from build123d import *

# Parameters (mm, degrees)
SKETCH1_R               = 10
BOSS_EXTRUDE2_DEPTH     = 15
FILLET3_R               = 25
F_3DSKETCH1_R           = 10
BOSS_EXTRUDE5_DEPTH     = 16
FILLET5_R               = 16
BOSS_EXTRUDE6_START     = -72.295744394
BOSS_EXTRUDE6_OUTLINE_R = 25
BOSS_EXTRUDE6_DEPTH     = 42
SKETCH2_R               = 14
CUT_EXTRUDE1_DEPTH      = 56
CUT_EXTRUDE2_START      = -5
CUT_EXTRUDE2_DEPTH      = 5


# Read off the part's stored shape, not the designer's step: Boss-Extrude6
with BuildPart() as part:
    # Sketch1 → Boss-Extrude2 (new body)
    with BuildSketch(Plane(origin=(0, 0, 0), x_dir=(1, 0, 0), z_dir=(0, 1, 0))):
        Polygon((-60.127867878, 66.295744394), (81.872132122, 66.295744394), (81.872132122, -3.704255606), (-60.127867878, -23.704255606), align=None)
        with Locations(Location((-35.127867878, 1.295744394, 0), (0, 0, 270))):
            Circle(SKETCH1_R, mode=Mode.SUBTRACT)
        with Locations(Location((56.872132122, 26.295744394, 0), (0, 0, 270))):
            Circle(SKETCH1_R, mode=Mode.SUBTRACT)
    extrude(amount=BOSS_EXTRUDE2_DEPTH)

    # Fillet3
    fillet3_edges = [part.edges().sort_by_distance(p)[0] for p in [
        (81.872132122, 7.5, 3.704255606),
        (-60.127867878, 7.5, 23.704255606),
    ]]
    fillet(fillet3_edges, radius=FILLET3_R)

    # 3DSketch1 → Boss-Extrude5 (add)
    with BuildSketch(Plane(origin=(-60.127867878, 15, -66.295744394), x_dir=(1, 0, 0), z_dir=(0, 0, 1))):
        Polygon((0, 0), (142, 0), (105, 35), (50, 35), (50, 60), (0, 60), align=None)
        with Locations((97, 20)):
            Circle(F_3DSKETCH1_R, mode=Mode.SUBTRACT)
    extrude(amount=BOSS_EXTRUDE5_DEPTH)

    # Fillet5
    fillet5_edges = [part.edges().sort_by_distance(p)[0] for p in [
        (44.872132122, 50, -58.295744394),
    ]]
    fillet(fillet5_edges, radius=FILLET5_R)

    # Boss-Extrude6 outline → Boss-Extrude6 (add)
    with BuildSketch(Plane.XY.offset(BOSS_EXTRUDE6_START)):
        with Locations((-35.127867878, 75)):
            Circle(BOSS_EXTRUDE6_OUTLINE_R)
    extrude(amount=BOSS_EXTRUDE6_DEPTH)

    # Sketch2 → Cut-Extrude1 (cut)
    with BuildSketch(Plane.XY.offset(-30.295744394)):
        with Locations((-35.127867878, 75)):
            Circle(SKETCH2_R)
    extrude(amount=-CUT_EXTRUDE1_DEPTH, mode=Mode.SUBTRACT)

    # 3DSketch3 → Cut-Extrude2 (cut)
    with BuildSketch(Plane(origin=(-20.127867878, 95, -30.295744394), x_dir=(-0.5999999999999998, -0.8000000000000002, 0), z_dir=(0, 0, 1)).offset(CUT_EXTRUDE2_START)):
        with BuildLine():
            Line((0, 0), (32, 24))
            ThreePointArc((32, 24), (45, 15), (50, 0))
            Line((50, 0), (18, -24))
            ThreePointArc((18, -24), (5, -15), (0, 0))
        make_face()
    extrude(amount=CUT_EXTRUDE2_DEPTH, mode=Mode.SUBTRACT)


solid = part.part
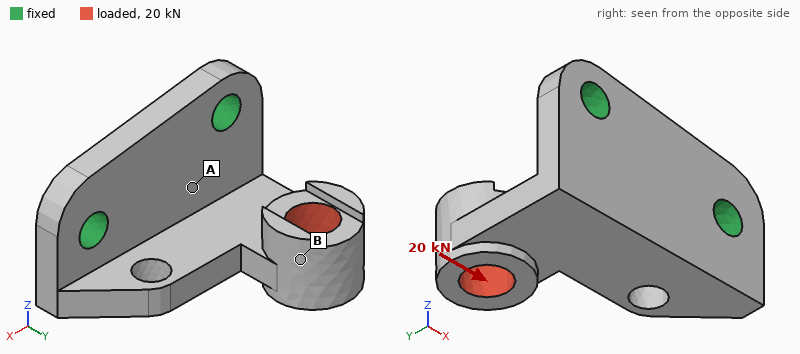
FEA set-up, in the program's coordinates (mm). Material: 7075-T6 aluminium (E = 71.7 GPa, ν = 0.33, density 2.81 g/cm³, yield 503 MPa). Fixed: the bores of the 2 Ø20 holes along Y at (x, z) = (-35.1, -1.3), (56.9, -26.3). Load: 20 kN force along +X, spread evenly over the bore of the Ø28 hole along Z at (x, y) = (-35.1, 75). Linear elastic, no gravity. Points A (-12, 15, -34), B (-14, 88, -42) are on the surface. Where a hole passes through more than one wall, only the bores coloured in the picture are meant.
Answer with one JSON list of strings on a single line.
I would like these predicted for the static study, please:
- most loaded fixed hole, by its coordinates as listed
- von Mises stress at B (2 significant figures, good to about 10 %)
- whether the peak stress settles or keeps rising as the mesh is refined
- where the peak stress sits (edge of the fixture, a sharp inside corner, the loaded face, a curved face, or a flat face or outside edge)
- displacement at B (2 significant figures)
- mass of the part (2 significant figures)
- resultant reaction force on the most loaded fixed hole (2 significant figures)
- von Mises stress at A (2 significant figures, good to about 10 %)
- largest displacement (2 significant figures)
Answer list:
["(56.9, -26.3)", "28 MPa", "keeps rising", "edge of the fixture", "0.73 mm", "780 g", "20 kN", "93 MPa", "0.96 mm"]
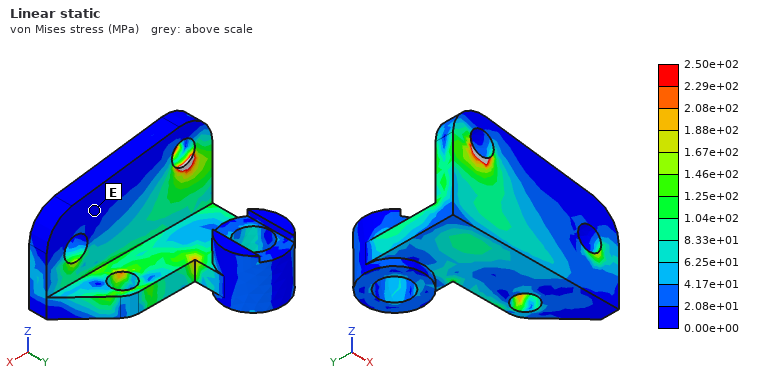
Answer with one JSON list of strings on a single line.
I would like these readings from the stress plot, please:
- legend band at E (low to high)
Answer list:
["0.00e+00 to 2.08e+01 MPa"]
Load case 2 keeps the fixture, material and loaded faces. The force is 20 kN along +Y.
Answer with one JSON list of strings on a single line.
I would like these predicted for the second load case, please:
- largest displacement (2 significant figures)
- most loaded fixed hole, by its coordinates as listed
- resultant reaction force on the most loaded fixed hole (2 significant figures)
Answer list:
["0.90 mm", "(-35.1, -1.3)", "17 kN"]
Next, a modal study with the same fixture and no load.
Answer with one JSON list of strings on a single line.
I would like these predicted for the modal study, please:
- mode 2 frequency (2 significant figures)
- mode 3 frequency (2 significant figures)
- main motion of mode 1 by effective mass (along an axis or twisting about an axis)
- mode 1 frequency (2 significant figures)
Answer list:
["2000 Hz", "3100 Hz", "along Z", "960 Hz"]
